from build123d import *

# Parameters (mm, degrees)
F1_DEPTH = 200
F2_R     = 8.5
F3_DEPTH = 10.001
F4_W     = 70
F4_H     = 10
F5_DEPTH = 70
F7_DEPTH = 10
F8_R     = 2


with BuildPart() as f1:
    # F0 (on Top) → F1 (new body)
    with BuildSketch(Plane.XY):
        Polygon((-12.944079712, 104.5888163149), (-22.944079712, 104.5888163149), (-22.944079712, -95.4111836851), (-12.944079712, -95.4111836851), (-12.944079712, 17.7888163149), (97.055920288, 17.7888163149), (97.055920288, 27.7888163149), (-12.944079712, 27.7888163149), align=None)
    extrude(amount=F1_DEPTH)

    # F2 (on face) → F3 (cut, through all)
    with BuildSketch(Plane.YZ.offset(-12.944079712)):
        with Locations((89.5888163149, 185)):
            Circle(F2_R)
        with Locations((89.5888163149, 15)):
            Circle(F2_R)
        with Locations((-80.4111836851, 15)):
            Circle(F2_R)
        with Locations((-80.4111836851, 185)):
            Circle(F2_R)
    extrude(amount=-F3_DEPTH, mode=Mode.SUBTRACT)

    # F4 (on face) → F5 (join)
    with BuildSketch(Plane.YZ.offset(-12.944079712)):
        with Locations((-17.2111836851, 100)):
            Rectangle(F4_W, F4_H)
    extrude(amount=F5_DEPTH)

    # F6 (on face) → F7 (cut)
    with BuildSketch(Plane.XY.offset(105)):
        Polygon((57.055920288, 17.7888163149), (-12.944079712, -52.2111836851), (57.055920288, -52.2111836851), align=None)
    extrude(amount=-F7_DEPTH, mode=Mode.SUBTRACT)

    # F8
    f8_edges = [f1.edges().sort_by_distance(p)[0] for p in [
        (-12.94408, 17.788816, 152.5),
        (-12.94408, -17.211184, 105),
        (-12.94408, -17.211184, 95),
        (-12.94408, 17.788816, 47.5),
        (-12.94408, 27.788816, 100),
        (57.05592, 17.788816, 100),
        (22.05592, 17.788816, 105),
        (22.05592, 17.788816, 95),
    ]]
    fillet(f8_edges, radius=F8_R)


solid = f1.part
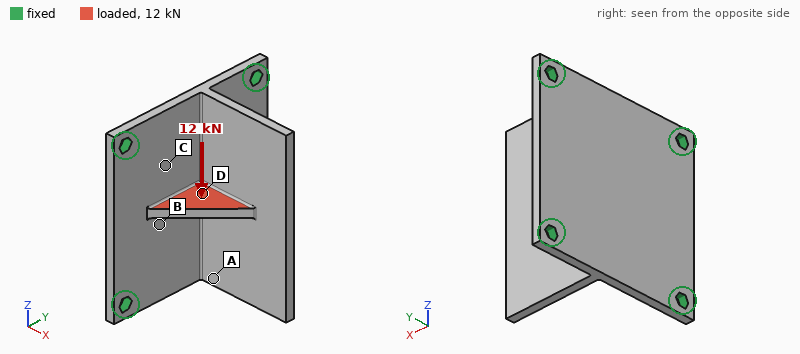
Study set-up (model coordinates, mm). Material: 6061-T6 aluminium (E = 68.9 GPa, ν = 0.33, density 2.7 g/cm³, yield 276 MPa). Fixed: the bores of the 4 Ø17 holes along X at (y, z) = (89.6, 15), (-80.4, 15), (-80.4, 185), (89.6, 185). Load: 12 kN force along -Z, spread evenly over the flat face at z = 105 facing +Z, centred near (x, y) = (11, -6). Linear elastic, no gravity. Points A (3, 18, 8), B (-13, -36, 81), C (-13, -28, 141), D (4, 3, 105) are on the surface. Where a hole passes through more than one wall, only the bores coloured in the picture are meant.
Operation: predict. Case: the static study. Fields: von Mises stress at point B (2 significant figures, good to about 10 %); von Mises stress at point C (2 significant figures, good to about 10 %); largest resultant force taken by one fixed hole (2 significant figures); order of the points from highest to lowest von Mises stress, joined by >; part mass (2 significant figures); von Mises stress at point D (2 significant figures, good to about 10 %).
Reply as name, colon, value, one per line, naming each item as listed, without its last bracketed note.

von Mises stress at point B: 25 MPa
von Mises stress at point C: 15 MPa
largest resultant force taken by one fixed hole: 3.8 kN
order of the points from highest to lowest von Mises stress, joined by >: D > B > C > A
part mass: 1.7 kg
von Mises stress at point D: 36 MPa
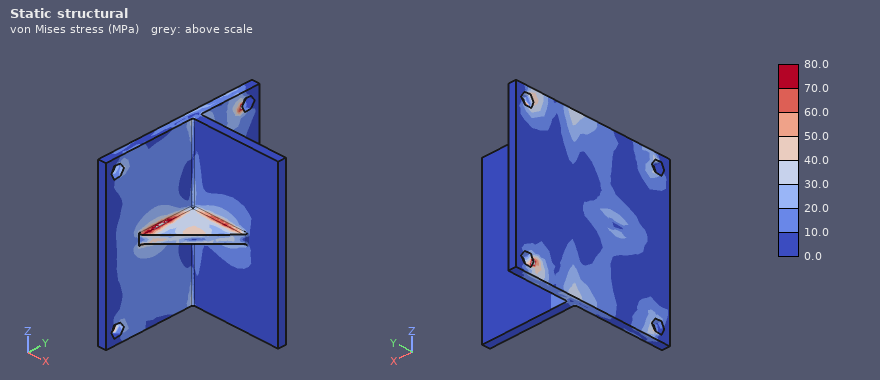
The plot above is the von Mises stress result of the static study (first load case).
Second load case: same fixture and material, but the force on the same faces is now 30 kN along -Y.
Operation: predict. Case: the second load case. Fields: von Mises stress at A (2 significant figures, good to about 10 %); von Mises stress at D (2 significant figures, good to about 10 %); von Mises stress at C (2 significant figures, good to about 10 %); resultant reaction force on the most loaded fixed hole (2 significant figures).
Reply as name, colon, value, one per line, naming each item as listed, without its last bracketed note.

von Mises stress at A: 40 MPa
von Mises stress at D: 63 MPa
von Mises stress at C: 55 MPa
resultant reaction force on the most loaded fixed hole: 9.3 kN
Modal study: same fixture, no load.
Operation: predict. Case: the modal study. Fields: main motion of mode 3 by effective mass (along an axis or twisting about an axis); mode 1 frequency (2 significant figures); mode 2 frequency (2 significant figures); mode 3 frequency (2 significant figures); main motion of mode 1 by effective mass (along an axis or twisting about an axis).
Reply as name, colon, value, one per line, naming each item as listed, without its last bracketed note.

main motion of mode 3 by effective mass: along X
mode 1 frequency: 870 Hz
mode 2 frequency: 970 Hz
mode 3 frequency: 1000 Hz
main motion of mode 1 by effective mass: along Y
